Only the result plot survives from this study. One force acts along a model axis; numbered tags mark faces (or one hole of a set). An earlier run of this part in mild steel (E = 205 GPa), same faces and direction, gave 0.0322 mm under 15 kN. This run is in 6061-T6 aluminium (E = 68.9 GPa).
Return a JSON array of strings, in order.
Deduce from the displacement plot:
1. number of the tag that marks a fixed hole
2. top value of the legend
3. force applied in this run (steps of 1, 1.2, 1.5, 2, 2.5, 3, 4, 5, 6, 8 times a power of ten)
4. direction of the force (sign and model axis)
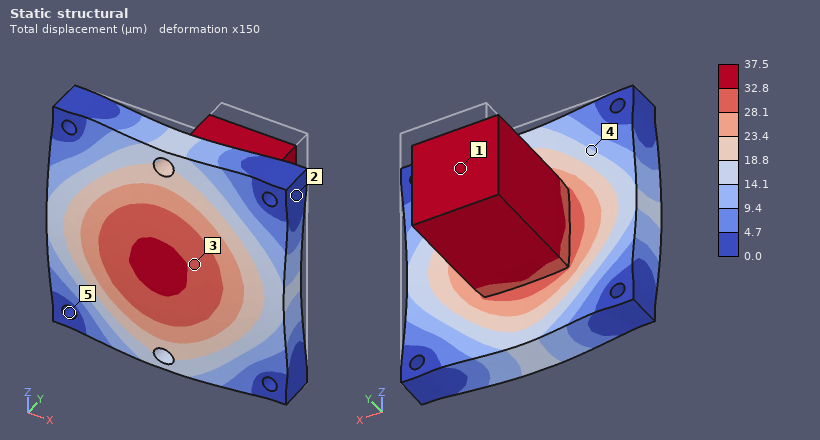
["5", "37.5 µm", "6 kN", "-Y"]
